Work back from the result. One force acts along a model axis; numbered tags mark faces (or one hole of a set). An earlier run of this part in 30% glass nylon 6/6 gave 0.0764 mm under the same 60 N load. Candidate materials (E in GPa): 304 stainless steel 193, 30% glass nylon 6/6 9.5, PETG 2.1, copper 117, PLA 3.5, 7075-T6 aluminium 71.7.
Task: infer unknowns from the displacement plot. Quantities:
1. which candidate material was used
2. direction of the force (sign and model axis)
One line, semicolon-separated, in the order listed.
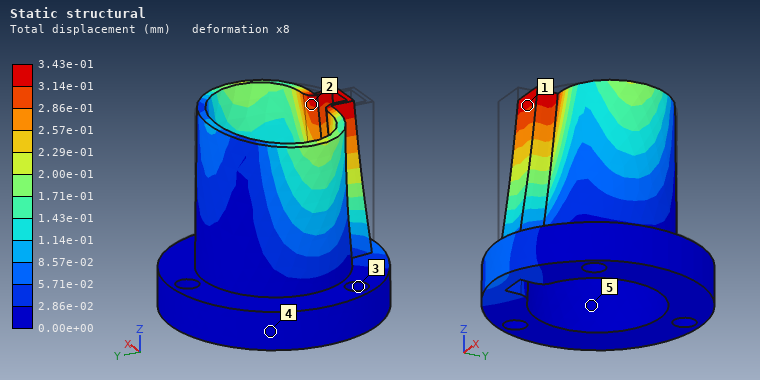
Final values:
PETG; +Y
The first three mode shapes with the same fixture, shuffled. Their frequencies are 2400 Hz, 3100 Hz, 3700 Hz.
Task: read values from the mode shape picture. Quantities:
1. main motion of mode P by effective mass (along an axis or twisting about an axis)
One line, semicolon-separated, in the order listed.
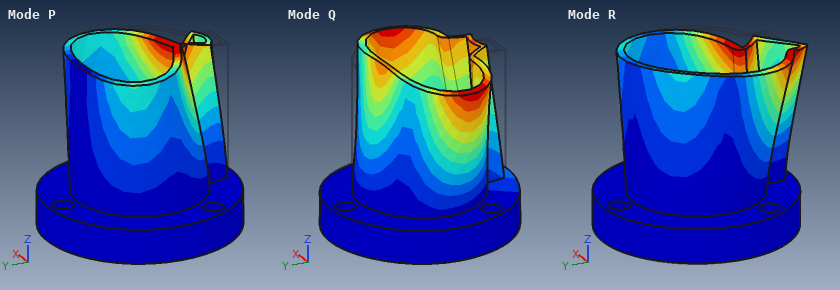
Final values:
along Y
